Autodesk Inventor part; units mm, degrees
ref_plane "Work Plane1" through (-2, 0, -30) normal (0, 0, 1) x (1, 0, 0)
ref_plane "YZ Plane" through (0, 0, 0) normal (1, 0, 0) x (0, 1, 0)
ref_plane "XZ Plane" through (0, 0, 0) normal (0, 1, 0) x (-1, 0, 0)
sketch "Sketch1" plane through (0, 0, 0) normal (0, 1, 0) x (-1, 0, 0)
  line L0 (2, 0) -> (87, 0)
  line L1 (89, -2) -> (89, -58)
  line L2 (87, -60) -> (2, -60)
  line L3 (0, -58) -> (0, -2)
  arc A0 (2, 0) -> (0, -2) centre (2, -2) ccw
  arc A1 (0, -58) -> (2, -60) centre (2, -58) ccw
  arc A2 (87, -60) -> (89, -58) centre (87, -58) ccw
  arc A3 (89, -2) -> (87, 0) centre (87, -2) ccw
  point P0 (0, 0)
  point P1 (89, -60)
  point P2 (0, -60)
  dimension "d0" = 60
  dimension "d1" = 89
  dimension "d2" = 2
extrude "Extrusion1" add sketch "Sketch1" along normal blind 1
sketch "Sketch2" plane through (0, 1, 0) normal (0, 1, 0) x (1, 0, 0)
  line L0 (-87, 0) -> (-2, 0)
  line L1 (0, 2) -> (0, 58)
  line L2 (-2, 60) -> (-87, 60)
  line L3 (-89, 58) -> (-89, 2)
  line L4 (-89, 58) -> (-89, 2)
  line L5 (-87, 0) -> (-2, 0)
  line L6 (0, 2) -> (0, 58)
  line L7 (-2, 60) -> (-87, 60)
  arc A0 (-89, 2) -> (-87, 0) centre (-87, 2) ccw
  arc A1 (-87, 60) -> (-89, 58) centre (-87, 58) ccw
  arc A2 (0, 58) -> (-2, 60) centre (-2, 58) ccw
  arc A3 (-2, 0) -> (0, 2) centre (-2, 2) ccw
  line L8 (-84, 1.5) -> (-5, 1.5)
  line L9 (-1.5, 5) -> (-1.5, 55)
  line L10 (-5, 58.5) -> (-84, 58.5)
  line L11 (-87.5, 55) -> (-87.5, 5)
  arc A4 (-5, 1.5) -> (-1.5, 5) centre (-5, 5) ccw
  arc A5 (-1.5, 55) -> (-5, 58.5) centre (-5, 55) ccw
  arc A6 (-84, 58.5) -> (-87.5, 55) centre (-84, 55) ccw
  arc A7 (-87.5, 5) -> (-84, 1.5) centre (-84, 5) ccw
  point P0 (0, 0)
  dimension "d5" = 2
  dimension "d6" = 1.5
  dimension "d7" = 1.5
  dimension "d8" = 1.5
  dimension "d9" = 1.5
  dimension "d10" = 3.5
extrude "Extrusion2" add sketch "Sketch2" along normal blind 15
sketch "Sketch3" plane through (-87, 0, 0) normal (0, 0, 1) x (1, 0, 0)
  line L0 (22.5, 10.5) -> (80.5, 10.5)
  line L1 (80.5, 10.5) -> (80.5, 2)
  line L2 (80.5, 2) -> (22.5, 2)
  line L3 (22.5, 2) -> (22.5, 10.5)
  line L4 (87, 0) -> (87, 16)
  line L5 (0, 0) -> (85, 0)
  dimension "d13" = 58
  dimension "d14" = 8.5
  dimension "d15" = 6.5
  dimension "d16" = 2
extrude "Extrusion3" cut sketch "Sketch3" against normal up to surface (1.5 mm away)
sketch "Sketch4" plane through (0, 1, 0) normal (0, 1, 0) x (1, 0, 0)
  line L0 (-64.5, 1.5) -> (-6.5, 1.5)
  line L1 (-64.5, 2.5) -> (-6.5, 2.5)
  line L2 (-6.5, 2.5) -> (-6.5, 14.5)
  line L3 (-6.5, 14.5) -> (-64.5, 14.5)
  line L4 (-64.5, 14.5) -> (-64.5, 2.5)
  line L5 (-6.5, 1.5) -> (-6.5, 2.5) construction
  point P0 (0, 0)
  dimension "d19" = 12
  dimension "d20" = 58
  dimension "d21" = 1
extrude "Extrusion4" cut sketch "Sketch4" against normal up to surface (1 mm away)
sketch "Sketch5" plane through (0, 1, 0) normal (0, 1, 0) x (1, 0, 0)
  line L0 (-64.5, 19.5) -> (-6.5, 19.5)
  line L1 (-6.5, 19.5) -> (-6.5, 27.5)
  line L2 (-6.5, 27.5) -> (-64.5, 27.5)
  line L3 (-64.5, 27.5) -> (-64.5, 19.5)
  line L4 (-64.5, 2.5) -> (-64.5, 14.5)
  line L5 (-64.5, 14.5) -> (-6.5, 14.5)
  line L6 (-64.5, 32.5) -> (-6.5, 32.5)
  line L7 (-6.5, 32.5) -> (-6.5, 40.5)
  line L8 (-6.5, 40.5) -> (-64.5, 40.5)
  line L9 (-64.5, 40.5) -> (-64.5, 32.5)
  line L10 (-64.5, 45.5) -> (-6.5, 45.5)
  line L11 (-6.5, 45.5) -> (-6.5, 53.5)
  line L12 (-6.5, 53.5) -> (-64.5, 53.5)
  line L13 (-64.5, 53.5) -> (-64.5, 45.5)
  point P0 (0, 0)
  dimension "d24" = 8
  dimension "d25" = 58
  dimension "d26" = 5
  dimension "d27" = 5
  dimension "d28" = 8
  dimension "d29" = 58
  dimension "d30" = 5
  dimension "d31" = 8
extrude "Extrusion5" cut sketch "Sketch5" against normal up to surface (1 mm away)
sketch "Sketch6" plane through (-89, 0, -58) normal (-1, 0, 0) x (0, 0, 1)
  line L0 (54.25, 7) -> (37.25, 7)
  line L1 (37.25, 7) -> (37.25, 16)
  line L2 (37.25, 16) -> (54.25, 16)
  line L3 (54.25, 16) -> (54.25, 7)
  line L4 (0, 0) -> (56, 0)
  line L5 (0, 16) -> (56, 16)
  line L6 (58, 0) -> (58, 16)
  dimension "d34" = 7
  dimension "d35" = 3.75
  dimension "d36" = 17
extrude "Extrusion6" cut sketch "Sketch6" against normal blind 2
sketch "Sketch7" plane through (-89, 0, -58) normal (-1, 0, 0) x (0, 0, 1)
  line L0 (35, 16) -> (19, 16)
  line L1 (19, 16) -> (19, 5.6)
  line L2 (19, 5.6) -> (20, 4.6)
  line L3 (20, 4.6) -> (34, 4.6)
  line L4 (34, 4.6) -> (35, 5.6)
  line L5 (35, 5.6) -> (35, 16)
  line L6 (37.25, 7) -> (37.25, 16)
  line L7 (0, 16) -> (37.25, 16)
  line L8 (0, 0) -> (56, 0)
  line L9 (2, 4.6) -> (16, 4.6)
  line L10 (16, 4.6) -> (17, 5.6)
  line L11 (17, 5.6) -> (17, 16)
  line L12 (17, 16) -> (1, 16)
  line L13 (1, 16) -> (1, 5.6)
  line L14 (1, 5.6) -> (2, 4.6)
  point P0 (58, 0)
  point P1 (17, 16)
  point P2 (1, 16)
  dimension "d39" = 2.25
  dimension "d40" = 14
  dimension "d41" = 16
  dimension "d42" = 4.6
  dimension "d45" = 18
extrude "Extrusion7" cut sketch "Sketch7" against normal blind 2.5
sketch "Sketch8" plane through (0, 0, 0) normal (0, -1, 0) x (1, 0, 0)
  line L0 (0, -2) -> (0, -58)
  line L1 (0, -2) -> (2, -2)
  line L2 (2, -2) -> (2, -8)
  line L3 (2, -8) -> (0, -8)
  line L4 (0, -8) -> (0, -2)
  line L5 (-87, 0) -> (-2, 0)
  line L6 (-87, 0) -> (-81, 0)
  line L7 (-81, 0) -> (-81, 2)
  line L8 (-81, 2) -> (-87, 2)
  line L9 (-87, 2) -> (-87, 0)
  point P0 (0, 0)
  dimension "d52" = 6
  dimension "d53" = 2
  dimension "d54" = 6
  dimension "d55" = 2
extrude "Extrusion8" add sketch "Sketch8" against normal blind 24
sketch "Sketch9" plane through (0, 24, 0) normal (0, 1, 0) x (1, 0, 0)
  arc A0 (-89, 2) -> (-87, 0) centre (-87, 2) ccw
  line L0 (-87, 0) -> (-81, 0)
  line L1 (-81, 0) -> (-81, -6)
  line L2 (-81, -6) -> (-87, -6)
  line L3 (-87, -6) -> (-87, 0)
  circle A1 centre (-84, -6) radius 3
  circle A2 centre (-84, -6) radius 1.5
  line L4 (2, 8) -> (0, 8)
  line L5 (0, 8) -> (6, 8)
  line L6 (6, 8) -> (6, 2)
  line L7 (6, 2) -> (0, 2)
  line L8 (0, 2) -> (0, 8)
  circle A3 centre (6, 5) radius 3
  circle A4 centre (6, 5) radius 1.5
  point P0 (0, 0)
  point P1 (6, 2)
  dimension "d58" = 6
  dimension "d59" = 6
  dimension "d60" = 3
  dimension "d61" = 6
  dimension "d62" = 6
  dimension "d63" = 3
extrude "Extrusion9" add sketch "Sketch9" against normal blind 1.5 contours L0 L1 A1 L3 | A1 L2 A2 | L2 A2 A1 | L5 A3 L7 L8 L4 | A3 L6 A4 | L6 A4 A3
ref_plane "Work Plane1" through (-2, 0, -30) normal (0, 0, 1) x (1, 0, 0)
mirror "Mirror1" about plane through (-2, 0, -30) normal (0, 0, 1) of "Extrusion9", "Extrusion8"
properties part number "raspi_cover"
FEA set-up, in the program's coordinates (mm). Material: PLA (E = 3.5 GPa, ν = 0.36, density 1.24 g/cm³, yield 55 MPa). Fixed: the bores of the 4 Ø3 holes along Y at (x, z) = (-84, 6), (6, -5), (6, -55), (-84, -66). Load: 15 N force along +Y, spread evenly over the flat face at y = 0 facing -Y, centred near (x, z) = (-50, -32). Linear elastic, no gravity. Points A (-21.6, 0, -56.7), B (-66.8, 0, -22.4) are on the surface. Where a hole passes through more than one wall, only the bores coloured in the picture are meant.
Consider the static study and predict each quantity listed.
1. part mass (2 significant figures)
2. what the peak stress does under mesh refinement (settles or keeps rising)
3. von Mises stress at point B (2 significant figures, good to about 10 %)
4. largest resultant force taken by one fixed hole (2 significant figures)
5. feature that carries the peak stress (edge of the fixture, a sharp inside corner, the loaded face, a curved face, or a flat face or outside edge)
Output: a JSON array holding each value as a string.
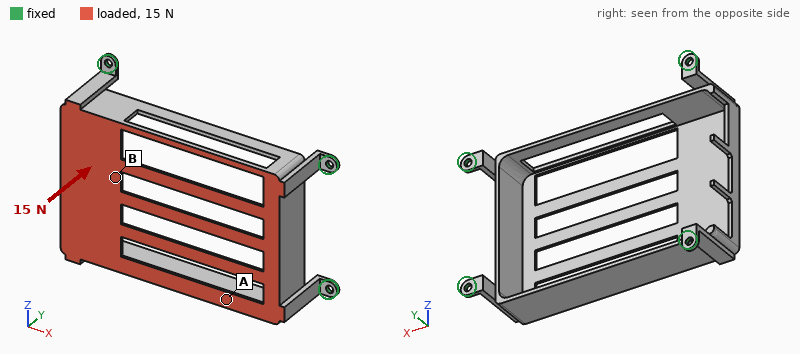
["12 g", "keeps rising", "4.2 MPa", "5.5 N", "a sharp inside corner"]
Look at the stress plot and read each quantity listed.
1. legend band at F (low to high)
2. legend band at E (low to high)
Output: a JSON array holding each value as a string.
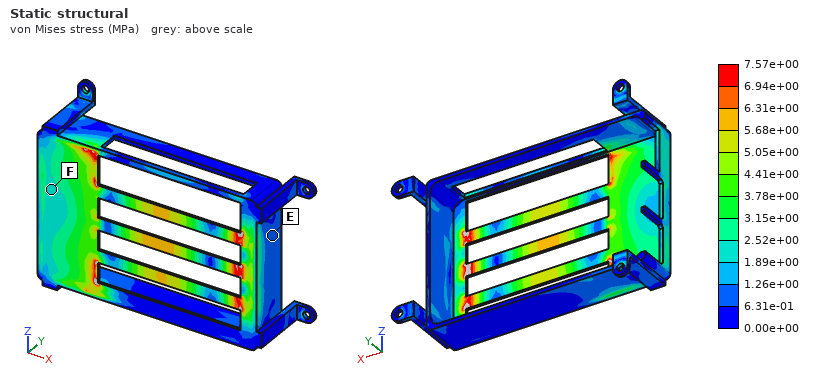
["1.89e+00 to 2.52e+00 MPa", "6.31e-01 to 1.26e+00 MPa"]
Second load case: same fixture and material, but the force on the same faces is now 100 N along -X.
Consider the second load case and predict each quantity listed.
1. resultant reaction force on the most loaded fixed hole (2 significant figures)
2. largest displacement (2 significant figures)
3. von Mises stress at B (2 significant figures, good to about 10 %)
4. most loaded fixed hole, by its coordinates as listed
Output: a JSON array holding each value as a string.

["43 N", "0.83 mm", "2.8 MPa", "(-84, -66)"]
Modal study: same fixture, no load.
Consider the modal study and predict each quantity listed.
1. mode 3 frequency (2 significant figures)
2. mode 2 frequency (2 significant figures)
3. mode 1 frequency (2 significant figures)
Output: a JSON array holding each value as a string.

["420 Hz", "390 Hz", "330 Hz"]
